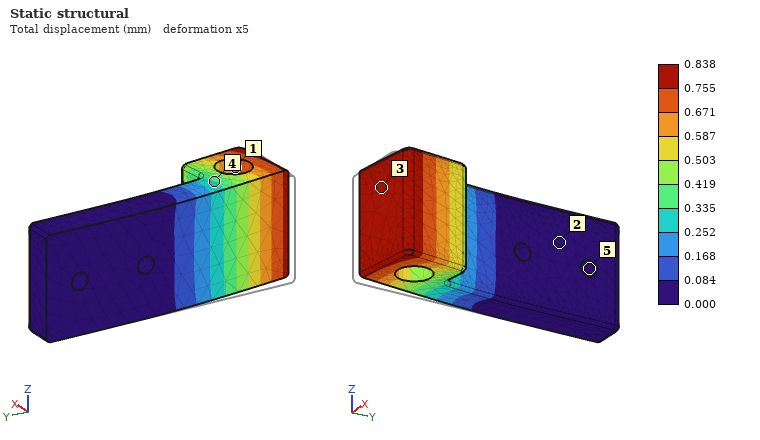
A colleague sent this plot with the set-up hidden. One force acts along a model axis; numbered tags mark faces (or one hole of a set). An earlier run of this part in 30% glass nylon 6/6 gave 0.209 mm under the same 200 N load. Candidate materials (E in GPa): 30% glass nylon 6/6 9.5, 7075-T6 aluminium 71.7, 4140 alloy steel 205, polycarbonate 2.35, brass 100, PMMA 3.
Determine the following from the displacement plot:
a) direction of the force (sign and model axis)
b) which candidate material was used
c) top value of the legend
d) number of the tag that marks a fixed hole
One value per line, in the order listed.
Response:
+X
polycarbonate
0.838 mm
5
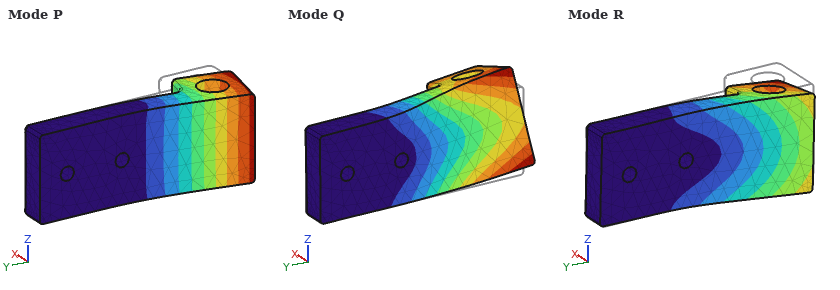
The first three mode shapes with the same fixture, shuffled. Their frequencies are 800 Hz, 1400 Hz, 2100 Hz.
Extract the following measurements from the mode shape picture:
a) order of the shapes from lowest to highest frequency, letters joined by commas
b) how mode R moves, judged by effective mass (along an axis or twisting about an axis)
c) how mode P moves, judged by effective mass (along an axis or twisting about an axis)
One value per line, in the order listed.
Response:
P, R, Q
along Z
along X
